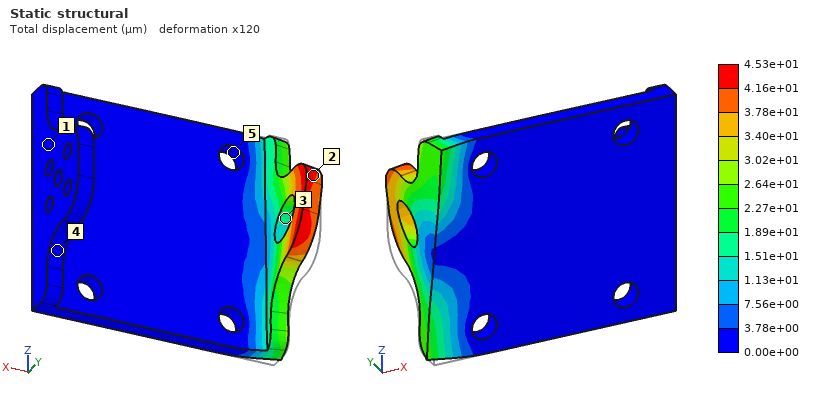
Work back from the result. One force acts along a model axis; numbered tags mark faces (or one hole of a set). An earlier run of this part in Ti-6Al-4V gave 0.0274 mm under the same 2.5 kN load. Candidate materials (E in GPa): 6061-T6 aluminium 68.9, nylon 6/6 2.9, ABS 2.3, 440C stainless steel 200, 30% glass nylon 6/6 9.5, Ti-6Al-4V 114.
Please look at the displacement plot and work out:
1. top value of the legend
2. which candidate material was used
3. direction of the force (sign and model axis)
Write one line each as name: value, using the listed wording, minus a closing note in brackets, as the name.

top value of the legend: 4.53e+01 µm
which candidate material was used: 6061-T6 aluminium
direction of the force: +Z
